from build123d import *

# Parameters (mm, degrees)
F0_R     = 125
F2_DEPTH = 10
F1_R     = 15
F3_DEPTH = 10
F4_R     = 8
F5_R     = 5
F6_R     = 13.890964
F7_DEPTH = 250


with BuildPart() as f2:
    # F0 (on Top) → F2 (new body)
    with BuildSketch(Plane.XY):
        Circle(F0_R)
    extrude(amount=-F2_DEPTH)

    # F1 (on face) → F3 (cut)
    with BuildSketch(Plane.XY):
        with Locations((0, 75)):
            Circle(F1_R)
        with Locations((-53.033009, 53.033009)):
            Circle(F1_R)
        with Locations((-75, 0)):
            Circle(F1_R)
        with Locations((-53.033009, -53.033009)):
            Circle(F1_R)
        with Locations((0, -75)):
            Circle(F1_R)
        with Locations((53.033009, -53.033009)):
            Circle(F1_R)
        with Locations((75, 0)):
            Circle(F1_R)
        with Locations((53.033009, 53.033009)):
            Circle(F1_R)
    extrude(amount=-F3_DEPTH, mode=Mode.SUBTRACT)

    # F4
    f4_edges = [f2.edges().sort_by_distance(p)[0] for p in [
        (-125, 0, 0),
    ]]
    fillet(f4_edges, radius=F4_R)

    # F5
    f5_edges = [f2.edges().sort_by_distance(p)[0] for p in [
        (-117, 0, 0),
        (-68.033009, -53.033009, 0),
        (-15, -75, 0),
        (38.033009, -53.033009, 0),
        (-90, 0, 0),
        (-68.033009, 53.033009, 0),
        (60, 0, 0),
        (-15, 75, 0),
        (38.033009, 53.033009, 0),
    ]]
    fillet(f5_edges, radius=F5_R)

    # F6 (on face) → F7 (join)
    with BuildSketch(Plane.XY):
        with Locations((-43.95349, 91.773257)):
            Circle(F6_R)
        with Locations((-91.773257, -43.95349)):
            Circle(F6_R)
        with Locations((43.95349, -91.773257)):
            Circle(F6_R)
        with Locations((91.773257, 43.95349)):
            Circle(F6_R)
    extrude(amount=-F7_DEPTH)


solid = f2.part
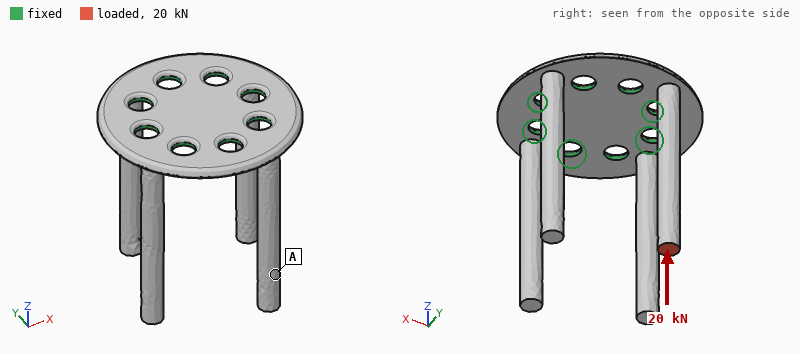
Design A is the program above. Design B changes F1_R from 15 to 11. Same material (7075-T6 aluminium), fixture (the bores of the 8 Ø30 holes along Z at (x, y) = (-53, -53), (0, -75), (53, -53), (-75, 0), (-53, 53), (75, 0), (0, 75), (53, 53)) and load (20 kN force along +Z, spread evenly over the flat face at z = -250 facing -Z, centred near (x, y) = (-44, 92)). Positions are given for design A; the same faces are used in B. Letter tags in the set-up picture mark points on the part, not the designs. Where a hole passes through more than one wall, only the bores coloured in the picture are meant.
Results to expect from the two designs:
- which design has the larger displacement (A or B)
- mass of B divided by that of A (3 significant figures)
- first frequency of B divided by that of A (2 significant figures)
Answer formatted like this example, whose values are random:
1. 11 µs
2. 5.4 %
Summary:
1. B
2. 1.03
3. 0.96
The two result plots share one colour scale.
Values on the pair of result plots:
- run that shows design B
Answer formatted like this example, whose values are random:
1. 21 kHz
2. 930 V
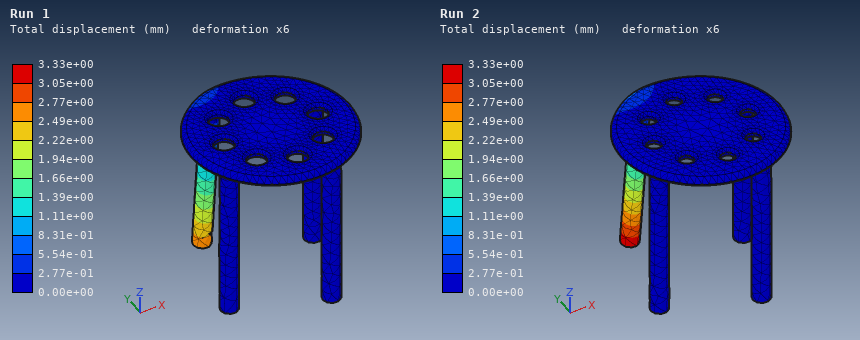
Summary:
1. Run 2
